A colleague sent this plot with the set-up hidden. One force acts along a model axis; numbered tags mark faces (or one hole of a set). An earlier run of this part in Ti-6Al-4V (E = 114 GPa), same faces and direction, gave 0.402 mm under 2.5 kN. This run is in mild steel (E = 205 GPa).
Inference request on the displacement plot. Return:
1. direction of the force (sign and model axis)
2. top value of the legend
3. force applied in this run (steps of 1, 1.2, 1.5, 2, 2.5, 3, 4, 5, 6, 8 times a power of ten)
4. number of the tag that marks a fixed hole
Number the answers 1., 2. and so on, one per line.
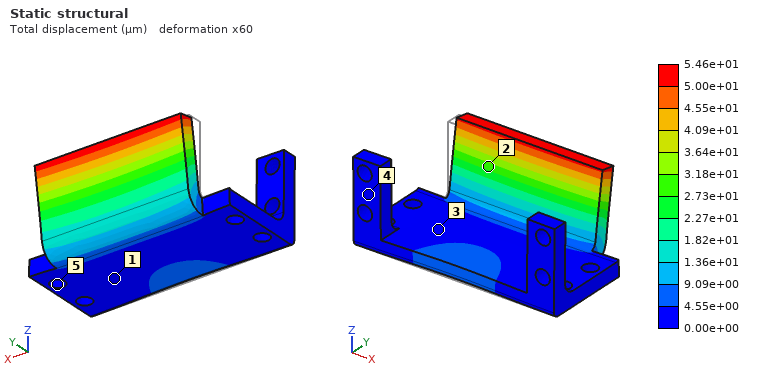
1. +Y
2. 5.46e+01 µm
3. 600 N
4. 5
